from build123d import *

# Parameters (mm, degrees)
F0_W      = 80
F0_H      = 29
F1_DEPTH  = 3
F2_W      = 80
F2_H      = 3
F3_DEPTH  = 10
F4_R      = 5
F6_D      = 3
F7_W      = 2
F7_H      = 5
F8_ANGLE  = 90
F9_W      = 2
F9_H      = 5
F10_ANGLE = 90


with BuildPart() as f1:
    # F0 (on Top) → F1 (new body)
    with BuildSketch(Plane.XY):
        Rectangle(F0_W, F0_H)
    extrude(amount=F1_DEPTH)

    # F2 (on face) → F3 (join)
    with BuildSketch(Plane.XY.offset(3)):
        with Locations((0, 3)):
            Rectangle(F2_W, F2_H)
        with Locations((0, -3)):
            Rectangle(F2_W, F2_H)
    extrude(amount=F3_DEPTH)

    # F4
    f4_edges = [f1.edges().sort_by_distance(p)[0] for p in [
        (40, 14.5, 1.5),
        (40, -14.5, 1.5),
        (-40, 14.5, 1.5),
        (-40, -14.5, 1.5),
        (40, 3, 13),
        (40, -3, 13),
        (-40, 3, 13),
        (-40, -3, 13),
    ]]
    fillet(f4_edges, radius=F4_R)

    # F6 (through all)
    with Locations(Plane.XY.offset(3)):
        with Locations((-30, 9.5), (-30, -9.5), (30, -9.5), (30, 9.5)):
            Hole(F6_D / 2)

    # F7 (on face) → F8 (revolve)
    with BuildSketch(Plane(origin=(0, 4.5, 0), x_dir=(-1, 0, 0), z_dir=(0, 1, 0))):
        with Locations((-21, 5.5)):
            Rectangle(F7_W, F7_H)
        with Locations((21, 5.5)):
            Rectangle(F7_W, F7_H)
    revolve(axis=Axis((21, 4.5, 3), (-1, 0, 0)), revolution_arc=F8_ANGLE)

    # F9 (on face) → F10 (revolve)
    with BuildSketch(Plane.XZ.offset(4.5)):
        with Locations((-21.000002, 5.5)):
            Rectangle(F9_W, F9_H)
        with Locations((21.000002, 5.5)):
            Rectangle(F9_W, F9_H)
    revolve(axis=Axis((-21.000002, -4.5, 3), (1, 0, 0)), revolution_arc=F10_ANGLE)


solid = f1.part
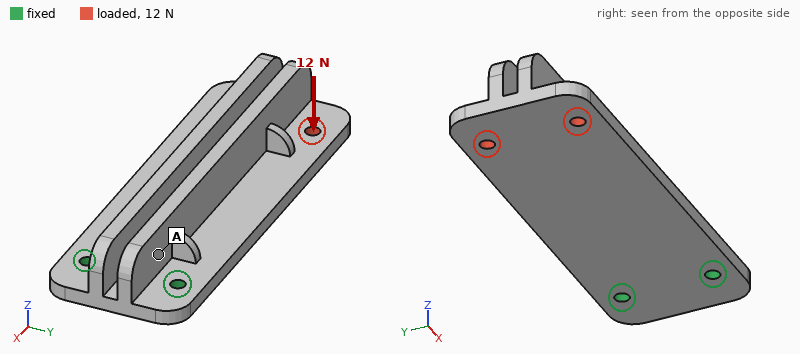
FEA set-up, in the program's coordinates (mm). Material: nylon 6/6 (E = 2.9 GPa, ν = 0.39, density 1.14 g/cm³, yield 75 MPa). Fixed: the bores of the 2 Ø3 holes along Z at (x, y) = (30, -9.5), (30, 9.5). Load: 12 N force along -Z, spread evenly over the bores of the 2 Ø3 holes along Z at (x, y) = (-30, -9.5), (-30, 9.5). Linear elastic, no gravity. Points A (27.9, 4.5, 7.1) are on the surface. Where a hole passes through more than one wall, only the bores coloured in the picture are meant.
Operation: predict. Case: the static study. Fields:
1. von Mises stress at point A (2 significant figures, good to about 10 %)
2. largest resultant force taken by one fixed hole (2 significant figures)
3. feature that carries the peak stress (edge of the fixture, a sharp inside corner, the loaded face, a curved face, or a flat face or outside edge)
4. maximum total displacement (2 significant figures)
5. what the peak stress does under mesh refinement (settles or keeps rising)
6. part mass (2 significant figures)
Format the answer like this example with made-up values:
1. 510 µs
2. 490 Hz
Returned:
1. 2.3 MPa
2. 9.3 N
3. edge of the fixture
4. 0.87 mm
5. keeps rising
6. 13 g
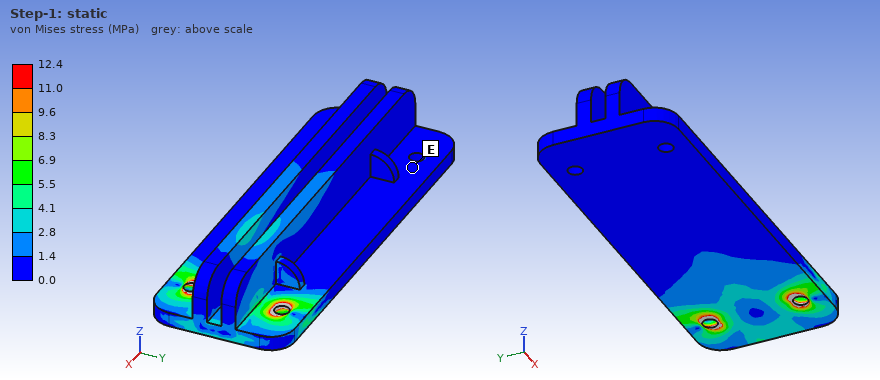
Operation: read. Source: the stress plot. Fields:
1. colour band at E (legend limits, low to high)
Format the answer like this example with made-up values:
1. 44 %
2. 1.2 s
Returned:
1. 0.0 to 1.4 MPa
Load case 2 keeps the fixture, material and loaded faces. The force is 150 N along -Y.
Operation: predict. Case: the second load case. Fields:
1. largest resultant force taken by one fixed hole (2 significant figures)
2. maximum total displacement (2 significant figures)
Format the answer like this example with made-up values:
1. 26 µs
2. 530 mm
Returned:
1. 450 N
2. 0.90 mm
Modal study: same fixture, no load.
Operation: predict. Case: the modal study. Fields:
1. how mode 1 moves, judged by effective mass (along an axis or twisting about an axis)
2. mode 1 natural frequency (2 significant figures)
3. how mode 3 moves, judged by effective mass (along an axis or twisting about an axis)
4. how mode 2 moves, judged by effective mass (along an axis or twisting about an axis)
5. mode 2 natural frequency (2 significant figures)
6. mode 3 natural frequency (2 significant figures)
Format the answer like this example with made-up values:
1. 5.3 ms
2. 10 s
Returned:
1. along Z
2. 280 Hz
3. along Y
4. along Y
5. 820 Hz
6. 1200 Hz
